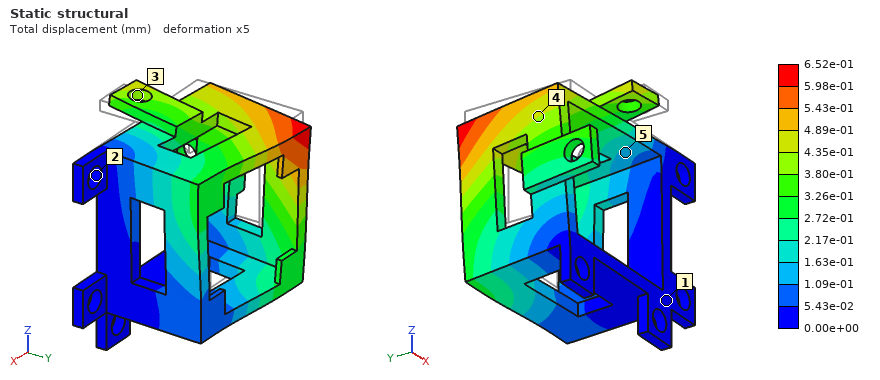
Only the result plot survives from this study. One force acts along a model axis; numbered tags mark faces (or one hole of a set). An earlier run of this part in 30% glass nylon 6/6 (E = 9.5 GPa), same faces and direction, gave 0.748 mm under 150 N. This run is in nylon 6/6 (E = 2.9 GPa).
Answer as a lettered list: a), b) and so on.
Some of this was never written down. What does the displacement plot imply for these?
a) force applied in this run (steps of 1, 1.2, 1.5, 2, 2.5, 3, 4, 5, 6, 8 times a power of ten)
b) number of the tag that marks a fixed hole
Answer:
a) 40 N
b) 2
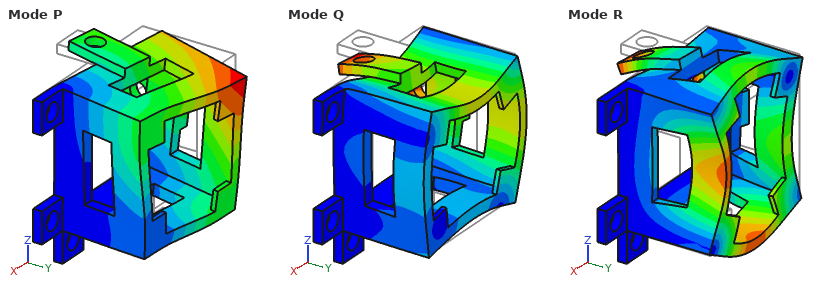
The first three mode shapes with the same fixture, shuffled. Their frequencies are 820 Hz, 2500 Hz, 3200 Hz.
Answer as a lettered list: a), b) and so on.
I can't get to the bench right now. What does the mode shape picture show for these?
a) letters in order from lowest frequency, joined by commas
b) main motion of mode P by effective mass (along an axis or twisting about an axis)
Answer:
a) P, Q, R
b) along Y
